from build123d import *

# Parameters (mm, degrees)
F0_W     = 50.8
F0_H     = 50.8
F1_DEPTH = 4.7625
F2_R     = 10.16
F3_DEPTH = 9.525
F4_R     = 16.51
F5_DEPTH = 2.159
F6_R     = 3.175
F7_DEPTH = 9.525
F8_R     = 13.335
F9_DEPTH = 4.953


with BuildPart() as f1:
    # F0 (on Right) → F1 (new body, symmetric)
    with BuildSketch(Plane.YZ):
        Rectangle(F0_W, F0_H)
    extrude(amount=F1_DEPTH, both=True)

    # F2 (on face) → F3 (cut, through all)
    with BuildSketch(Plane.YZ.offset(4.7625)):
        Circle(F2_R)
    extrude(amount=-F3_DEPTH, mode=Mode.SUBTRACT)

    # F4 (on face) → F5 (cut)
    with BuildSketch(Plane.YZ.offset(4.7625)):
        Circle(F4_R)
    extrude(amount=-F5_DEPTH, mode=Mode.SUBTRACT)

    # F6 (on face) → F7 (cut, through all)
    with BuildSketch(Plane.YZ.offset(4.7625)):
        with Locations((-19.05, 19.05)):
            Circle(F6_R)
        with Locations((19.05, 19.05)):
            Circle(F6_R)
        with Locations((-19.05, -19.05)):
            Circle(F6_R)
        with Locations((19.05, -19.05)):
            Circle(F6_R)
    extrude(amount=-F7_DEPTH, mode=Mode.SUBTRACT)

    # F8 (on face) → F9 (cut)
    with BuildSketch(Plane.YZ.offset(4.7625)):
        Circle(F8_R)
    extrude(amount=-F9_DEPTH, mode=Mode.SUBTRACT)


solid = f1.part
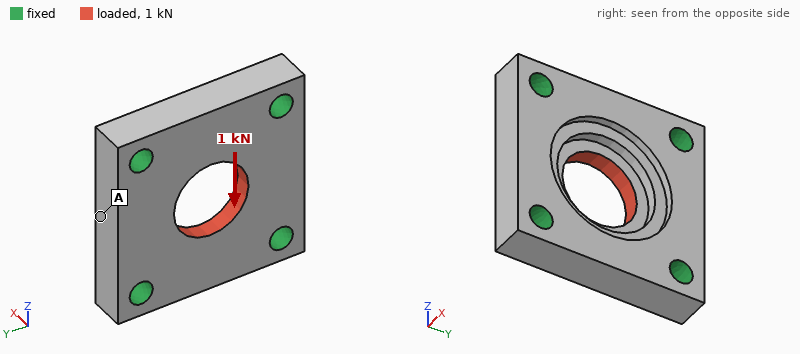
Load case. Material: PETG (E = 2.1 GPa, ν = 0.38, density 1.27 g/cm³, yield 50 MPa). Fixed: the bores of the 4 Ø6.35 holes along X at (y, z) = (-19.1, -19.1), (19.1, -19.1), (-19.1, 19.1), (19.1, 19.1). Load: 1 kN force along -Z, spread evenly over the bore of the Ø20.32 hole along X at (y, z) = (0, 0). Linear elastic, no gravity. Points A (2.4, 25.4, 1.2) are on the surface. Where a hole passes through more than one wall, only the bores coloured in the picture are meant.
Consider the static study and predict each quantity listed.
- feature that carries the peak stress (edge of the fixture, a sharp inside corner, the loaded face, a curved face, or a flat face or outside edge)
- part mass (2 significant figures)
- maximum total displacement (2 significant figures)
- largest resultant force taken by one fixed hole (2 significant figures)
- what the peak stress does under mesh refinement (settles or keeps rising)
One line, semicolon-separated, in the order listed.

edge of the fixture; 23 g; 48 µm; 270 N; keeps rising
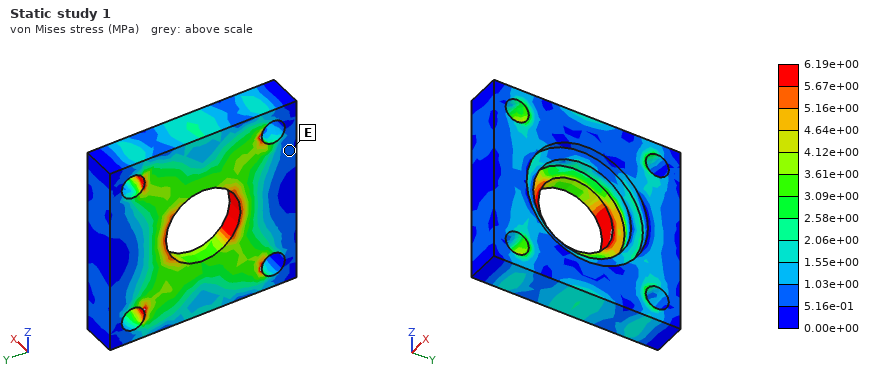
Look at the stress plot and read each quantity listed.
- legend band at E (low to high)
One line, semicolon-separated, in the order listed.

5.16e-01 to 1.03e+00 MPa
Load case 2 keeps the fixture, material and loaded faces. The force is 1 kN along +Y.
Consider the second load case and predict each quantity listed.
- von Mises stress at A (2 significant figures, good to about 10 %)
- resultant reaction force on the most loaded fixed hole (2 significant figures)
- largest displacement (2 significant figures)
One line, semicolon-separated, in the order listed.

2.0 MPa; 270 N; 48 µm
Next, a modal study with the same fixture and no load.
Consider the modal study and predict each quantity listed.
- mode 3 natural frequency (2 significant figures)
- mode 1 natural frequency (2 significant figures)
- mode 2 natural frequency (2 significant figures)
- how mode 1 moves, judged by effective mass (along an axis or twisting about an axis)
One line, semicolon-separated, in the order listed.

7600 Hz; 6700 Hz; 7300 Hz; along X
